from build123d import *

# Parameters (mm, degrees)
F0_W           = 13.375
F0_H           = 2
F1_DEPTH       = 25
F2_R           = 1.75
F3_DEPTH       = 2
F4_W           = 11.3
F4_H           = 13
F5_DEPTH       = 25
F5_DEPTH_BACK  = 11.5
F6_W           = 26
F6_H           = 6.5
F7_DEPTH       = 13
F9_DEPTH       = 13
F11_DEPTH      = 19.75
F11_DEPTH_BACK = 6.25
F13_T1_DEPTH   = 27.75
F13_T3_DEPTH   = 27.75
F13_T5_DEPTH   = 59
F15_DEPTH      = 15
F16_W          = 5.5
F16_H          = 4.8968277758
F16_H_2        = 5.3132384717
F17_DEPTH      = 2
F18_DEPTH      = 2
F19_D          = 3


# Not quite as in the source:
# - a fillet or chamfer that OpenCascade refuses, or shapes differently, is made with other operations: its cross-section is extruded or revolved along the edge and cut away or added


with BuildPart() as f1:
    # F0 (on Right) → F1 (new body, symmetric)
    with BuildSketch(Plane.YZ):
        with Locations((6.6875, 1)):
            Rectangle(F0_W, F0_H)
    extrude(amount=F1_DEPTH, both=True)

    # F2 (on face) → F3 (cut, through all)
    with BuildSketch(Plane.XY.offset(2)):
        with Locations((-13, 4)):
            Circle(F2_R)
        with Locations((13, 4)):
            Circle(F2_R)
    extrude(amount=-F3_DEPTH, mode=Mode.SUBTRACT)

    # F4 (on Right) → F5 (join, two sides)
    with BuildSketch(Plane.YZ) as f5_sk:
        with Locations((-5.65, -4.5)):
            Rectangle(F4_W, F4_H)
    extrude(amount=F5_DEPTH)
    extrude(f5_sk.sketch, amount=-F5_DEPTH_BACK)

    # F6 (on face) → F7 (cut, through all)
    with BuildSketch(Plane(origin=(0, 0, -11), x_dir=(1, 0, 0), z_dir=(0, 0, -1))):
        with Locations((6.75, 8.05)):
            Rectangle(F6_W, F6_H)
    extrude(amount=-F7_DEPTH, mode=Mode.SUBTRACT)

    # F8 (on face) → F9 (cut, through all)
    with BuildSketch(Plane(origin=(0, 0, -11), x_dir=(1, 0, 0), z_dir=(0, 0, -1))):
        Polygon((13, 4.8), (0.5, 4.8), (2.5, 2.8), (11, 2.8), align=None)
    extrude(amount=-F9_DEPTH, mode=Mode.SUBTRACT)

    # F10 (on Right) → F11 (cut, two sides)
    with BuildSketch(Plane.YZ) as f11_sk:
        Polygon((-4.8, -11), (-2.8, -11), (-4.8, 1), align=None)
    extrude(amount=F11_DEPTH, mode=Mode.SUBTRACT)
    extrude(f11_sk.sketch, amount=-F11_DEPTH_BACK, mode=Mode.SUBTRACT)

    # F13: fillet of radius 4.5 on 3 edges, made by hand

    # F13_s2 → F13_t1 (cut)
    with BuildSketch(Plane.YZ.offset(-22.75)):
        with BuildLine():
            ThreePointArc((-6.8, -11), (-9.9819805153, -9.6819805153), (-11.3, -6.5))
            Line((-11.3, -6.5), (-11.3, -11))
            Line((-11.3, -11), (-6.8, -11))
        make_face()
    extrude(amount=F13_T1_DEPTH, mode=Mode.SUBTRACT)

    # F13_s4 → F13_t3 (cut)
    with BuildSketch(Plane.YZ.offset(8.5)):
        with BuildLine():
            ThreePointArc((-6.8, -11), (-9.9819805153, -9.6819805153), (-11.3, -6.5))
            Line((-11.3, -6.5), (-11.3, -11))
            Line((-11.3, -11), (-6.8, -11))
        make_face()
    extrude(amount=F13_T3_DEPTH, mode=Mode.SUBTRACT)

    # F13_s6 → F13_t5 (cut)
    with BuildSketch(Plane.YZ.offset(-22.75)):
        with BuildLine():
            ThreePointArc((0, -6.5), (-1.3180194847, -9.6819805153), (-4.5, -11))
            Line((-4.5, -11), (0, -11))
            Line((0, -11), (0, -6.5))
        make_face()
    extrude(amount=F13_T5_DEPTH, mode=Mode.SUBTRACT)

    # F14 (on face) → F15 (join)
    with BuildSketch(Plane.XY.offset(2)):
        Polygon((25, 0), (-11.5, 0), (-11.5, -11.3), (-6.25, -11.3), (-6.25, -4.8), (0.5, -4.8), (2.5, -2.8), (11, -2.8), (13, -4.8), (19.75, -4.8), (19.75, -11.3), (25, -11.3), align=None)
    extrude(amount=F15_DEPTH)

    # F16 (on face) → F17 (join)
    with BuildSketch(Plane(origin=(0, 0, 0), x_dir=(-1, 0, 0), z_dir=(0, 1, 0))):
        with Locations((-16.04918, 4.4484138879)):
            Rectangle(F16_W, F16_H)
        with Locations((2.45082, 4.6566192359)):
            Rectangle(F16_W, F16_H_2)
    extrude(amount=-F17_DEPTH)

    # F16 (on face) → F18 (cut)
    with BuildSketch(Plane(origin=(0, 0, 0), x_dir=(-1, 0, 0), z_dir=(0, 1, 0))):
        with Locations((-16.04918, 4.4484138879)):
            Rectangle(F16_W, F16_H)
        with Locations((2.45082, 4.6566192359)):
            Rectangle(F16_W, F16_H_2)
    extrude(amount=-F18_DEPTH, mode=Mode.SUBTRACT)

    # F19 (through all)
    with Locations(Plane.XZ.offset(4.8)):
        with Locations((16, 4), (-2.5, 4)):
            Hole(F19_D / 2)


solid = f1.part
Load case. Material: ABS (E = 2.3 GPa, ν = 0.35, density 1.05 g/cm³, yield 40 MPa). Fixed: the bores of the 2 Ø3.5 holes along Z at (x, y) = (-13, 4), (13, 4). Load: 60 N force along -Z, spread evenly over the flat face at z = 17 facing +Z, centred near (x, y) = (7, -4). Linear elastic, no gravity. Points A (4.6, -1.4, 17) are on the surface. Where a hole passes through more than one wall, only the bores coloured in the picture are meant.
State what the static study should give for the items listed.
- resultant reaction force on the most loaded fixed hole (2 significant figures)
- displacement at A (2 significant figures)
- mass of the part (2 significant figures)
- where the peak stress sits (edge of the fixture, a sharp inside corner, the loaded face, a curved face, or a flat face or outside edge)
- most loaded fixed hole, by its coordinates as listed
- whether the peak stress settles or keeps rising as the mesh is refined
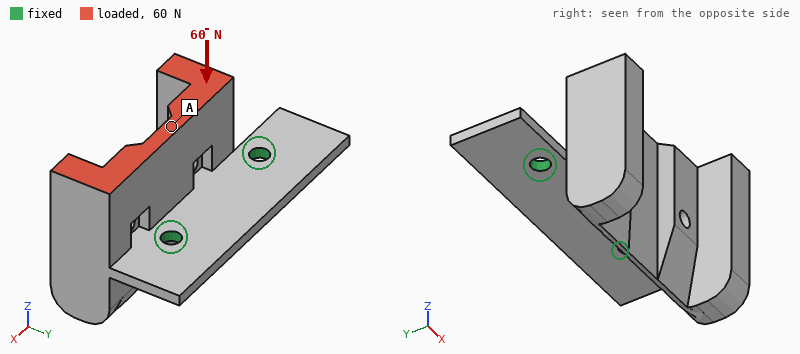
45 N
0.47 mm
7.3 g
edge of the fixture
(13, 4)
keeps rising
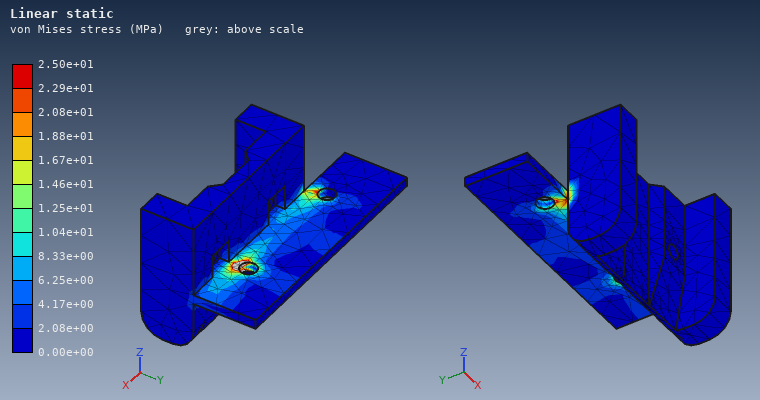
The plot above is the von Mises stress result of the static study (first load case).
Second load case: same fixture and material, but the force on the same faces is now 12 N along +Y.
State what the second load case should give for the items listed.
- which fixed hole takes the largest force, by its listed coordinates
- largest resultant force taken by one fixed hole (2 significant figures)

(13, 4)
8.8 N
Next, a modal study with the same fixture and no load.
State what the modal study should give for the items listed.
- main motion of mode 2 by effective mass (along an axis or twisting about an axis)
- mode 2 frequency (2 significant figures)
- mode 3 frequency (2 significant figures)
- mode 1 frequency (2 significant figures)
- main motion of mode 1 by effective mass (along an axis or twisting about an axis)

twisting about Y
1600 Hz
2700 Hz
660 Hz
along Z
